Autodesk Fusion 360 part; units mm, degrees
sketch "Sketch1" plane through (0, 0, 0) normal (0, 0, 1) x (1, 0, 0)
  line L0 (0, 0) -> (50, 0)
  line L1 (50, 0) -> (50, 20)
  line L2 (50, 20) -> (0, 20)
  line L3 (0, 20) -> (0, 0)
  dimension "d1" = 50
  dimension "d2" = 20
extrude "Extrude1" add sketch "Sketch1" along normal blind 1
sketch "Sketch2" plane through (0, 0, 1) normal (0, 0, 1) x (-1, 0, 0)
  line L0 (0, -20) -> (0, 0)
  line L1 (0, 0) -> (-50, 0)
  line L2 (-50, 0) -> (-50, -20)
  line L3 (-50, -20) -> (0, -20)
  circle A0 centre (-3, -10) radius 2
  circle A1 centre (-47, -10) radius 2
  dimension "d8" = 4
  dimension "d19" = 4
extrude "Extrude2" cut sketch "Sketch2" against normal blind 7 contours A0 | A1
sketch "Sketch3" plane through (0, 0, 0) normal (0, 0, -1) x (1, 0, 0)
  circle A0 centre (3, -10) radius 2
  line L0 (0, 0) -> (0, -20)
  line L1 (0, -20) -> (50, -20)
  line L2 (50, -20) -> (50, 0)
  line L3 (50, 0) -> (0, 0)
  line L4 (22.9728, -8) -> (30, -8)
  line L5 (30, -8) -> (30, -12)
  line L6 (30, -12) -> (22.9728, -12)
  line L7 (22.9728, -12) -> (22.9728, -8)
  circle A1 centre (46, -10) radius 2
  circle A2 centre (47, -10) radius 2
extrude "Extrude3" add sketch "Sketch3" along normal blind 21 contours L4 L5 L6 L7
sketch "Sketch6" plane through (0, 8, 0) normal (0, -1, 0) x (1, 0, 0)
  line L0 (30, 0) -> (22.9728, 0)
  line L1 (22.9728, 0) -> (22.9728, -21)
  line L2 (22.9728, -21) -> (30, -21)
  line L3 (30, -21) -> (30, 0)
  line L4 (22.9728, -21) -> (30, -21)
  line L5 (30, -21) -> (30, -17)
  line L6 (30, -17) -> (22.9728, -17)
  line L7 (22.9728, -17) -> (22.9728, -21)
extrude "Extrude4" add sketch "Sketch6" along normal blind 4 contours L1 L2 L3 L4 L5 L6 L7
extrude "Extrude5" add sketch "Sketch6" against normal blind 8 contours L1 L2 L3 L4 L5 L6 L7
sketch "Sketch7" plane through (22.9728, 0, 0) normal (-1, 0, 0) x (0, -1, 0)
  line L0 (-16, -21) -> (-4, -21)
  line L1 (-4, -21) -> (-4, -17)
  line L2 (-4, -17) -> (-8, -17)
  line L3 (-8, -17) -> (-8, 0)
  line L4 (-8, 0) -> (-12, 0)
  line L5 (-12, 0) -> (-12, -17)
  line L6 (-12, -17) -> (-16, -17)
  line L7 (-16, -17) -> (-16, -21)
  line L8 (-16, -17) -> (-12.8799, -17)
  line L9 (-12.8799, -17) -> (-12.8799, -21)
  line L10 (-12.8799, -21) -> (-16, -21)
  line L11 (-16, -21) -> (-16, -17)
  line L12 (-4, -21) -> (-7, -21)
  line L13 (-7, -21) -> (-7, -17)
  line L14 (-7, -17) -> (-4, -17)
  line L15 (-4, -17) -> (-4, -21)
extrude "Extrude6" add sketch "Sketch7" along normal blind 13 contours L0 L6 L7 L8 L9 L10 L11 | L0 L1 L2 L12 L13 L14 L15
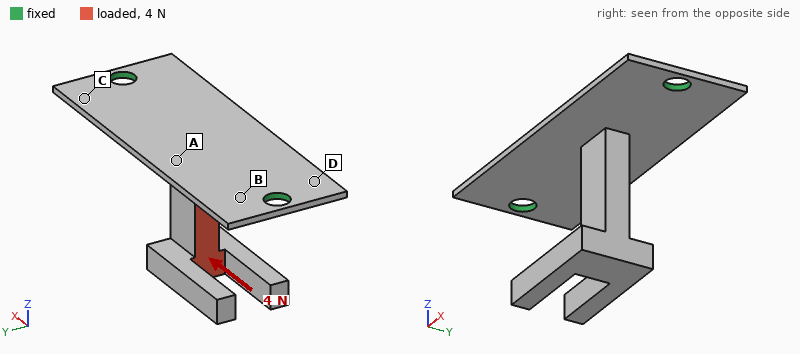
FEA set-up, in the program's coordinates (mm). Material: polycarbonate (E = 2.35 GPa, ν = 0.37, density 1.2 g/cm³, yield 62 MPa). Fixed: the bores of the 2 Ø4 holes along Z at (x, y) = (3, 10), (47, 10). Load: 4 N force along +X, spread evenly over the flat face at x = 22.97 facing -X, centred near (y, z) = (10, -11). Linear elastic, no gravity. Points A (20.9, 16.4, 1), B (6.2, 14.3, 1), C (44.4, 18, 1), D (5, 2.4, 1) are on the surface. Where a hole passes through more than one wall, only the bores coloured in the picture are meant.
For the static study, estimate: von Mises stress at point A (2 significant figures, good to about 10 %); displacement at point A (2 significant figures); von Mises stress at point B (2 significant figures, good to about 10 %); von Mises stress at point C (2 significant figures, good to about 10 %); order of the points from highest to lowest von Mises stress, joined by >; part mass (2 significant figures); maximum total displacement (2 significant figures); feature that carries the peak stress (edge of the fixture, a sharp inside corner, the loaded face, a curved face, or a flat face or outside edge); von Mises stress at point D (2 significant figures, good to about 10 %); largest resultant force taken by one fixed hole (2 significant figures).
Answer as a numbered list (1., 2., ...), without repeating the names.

1. 3.5 MPa
2. 0.11 mm
3. 2.1 MPa
4. 0.59 MPa
5. A > B > D > C
6. 2.5 g
7. 0.60 mm
8. a flat face or outside edge
9. 1.3 MPa
10. 2.6 N
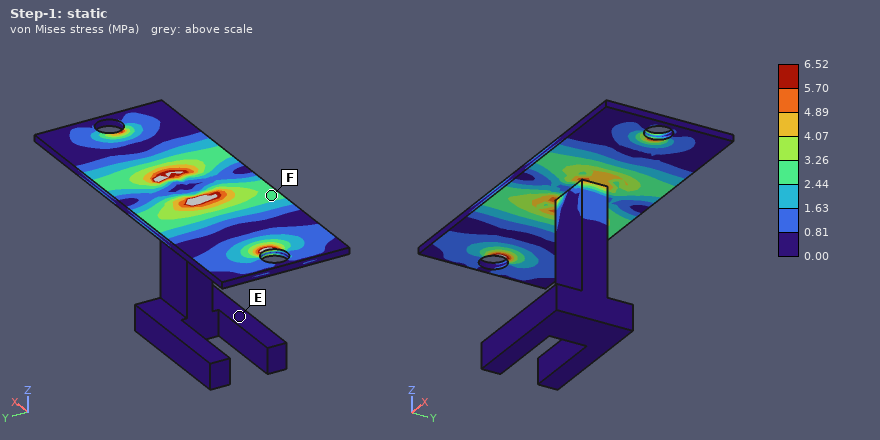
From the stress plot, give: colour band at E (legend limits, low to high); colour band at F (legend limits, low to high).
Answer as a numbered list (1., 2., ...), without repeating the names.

1. 0.00 to 0.81 MPa
2. 2.44 to 3.26 MPa
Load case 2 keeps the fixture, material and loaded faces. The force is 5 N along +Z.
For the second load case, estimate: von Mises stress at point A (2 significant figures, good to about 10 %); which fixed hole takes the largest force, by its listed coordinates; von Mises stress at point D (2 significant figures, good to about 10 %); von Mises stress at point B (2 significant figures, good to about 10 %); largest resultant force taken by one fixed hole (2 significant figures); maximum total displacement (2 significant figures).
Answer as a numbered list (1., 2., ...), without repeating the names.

1. 5.4 MPa
2. (3, 10)
3. 3.2 MPa
4. 5.0 MPa
5. 3.0 N
6. 0.64 mm
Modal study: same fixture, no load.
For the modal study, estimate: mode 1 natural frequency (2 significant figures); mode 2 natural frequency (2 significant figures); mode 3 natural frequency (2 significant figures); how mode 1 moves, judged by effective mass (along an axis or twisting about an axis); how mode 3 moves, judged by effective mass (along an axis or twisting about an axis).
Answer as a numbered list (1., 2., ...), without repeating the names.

1. 200 Hz
2. 340 Hz
3. 480 Hz
4. along Y
5. along Z
